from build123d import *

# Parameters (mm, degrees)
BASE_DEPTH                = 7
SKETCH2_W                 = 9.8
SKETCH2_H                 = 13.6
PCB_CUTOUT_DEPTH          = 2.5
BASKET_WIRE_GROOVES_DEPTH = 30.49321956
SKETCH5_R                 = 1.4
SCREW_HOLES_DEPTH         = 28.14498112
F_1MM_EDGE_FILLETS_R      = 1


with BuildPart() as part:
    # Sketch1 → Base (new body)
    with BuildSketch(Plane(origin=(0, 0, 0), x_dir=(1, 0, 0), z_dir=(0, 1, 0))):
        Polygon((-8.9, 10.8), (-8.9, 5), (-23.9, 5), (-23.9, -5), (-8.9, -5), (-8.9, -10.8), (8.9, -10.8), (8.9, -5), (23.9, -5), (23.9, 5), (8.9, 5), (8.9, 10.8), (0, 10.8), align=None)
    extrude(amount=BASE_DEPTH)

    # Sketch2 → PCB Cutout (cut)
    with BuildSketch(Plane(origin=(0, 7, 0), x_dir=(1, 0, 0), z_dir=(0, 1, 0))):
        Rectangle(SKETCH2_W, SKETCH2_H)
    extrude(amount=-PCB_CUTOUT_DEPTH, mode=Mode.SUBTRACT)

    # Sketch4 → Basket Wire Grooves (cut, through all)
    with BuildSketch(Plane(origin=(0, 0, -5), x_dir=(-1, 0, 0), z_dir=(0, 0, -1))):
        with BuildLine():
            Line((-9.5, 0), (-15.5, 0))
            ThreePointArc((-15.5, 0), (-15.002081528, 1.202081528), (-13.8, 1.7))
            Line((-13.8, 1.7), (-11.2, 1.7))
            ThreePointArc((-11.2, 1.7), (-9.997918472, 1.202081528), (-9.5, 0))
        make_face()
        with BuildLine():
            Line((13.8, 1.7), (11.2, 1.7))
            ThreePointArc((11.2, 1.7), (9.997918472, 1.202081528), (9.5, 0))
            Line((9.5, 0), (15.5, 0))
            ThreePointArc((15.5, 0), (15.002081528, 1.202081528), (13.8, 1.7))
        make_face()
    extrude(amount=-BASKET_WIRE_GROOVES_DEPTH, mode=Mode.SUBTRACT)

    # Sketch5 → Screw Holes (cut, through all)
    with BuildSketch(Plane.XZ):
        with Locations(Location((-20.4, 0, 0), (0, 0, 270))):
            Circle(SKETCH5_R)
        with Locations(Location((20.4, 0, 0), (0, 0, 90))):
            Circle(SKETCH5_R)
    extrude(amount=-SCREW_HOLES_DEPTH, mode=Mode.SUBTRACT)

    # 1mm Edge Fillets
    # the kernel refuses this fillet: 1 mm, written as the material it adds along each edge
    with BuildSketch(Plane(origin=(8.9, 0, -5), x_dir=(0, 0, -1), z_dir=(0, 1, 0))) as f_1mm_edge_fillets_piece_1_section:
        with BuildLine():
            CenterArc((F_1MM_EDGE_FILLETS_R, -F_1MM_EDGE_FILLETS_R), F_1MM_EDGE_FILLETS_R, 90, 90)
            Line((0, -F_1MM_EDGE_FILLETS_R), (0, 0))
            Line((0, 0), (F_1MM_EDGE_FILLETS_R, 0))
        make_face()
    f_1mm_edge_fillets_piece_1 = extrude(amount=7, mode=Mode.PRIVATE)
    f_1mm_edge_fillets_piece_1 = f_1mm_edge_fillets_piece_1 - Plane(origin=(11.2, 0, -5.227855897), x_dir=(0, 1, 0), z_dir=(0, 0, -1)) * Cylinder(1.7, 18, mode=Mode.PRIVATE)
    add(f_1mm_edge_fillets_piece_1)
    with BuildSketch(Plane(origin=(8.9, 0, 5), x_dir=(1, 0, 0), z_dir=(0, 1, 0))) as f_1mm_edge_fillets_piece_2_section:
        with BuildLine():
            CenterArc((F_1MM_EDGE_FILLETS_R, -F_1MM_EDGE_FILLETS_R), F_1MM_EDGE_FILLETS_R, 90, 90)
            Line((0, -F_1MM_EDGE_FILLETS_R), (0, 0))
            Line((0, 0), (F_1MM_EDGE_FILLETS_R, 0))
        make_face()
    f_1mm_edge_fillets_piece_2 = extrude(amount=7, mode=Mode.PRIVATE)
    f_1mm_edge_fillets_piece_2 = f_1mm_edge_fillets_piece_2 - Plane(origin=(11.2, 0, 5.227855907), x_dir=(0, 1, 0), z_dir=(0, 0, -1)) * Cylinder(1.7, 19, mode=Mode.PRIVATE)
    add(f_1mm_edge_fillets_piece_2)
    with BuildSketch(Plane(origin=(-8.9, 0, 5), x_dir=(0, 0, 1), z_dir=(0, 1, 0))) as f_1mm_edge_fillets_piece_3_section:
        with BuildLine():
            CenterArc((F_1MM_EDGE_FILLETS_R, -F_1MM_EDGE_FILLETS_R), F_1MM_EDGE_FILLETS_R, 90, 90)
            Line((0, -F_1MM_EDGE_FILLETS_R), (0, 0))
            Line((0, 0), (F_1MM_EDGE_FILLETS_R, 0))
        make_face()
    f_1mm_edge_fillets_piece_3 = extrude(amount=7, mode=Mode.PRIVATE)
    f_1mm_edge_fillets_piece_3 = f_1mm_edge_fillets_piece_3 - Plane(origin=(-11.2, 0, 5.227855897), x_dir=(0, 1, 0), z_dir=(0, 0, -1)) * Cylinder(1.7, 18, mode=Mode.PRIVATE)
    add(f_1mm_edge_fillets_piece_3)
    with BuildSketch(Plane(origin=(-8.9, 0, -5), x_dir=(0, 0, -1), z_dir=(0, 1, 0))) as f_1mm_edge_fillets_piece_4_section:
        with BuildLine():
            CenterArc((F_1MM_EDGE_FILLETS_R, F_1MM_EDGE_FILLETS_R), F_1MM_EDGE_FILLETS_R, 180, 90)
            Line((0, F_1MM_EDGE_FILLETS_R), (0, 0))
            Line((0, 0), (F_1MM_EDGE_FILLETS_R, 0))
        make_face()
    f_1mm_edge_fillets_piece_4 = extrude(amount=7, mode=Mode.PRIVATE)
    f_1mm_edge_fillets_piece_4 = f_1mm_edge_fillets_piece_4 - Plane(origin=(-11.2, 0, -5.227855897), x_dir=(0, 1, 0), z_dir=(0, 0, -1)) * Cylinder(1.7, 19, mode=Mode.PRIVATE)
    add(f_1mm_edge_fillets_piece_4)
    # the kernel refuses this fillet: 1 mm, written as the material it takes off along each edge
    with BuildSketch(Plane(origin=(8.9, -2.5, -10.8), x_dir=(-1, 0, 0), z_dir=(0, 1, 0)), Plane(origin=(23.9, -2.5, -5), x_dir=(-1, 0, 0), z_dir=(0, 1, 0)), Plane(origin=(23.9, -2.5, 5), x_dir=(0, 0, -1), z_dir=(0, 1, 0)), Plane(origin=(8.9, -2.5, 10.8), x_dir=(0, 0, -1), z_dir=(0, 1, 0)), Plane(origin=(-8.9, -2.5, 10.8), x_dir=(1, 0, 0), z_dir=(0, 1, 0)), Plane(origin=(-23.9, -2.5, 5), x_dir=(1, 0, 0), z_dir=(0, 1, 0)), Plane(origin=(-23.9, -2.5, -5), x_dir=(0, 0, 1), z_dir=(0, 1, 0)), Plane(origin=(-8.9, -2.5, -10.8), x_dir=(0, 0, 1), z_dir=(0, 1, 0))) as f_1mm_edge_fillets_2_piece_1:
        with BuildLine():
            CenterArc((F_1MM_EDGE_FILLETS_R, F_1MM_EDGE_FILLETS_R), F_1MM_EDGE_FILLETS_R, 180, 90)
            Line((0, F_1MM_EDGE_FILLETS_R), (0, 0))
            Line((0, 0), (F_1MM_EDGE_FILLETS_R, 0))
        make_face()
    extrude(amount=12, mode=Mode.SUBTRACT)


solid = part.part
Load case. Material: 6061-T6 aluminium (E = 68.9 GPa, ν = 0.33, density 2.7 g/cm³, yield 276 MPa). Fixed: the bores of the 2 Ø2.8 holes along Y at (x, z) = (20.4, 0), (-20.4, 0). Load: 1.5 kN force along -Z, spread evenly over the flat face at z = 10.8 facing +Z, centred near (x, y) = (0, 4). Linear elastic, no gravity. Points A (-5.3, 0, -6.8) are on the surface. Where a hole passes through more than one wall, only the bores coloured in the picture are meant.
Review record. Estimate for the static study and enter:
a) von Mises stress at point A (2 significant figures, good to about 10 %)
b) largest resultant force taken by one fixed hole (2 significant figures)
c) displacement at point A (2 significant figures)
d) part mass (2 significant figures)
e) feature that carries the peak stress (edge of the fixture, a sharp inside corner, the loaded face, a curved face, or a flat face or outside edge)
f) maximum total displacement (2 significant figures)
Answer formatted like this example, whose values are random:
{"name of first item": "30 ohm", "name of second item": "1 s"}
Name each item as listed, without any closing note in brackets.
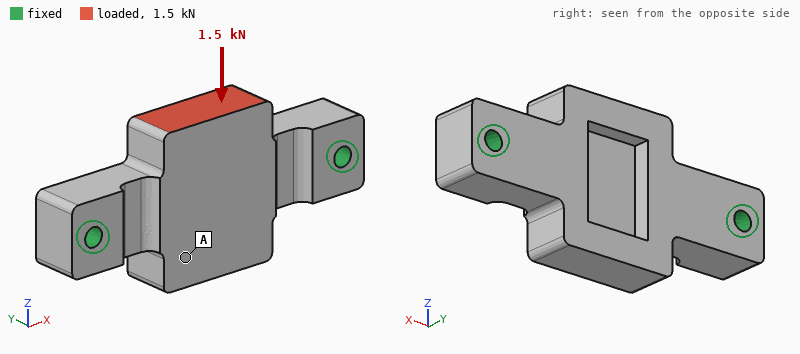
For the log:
{"von Mises stress at point A": "15 MPa", "largest resultant force taken by one fixed hole": "760 N", "displacement at point A": "19 µm", "part mass": "11 g", "feature that carries the peak stress": "a curved face", "maximum total displacement": "21 µm"}
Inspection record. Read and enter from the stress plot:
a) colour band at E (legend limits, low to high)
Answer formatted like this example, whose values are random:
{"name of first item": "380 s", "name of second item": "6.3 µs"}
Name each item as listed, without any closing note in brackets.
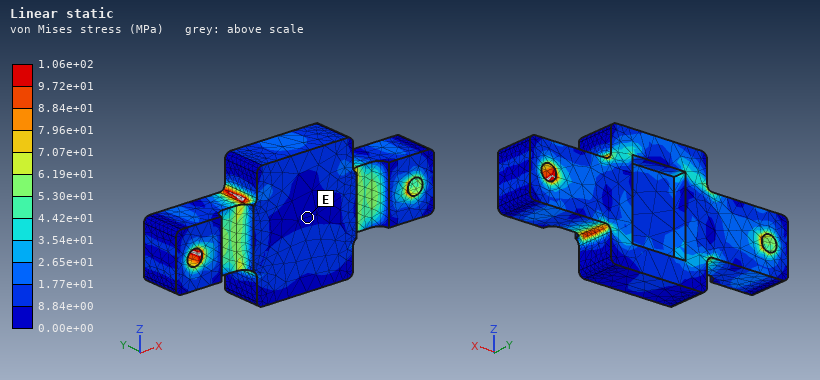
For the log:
{"colour band at E": "0.00e+00 to 8.84e+00 MPa"}
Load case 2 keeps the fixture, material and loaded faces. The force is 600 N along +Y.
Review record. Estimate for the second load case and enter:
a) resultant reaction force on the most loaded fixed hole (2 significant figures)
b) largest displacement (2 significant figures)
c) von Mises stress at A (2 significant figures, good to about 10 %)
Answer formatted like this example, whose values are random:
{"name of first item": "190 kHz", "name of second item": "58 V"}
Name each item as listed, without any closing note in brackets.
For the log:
{"resultant reaction force on the most loaded fixed hole": "370 N", "largest displacement": "63 µm", "von Mises stress at A": "11 MPa"}
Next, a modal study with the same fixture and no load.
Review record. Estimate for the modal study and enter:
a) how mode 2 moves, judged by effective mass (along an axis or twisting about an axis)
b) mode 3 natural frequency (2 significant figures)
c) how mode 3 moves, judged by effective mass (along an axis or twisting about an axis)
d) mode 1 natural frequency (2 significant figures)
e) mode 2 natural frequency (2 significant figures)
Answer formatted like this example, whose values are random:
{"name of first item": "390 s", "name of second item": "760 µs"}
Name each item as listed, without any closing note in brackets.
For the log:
{"how mode 2 moves, judged by effective mass": "along Y", "mode 3 natural frequency": "18 kHz", "how mode 3 moves, judged by effective mass": "along Z", "mode 1 natural frequency": "12 kHz", "mode 2 natural frequency": "13 kHz"}
